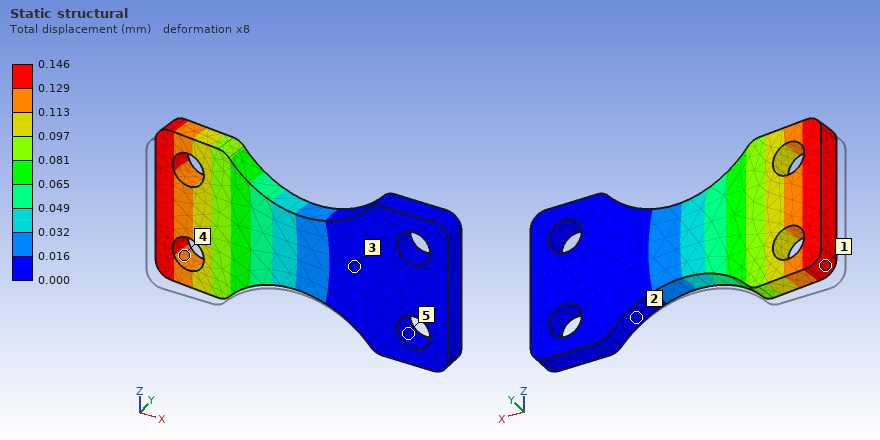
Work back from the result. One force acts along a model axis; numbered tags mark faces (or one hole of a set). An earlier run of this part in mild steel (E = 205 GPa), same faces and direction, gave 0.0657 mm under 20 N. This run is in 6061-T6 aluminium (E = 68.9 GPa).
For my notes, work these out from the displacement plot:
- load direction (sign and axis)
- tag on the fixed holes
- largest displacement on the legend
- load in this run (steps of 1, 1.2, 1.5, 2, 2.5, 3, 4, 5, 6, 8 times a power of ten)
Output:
+Y
5
0.146 mm
15 N
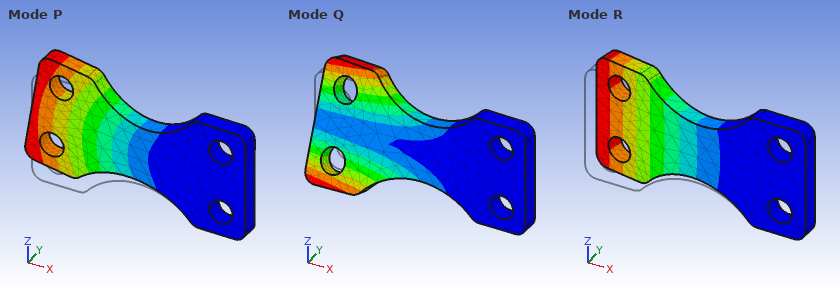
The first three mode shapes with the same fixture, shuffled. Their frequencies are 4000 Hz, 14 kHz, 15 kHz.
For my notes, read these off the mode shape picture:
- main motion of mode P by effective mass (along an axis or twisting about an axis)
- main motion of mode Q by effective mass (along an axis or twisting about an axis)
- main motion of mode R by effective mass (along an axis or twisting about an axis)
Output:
along Z
twisting about X
along Y
